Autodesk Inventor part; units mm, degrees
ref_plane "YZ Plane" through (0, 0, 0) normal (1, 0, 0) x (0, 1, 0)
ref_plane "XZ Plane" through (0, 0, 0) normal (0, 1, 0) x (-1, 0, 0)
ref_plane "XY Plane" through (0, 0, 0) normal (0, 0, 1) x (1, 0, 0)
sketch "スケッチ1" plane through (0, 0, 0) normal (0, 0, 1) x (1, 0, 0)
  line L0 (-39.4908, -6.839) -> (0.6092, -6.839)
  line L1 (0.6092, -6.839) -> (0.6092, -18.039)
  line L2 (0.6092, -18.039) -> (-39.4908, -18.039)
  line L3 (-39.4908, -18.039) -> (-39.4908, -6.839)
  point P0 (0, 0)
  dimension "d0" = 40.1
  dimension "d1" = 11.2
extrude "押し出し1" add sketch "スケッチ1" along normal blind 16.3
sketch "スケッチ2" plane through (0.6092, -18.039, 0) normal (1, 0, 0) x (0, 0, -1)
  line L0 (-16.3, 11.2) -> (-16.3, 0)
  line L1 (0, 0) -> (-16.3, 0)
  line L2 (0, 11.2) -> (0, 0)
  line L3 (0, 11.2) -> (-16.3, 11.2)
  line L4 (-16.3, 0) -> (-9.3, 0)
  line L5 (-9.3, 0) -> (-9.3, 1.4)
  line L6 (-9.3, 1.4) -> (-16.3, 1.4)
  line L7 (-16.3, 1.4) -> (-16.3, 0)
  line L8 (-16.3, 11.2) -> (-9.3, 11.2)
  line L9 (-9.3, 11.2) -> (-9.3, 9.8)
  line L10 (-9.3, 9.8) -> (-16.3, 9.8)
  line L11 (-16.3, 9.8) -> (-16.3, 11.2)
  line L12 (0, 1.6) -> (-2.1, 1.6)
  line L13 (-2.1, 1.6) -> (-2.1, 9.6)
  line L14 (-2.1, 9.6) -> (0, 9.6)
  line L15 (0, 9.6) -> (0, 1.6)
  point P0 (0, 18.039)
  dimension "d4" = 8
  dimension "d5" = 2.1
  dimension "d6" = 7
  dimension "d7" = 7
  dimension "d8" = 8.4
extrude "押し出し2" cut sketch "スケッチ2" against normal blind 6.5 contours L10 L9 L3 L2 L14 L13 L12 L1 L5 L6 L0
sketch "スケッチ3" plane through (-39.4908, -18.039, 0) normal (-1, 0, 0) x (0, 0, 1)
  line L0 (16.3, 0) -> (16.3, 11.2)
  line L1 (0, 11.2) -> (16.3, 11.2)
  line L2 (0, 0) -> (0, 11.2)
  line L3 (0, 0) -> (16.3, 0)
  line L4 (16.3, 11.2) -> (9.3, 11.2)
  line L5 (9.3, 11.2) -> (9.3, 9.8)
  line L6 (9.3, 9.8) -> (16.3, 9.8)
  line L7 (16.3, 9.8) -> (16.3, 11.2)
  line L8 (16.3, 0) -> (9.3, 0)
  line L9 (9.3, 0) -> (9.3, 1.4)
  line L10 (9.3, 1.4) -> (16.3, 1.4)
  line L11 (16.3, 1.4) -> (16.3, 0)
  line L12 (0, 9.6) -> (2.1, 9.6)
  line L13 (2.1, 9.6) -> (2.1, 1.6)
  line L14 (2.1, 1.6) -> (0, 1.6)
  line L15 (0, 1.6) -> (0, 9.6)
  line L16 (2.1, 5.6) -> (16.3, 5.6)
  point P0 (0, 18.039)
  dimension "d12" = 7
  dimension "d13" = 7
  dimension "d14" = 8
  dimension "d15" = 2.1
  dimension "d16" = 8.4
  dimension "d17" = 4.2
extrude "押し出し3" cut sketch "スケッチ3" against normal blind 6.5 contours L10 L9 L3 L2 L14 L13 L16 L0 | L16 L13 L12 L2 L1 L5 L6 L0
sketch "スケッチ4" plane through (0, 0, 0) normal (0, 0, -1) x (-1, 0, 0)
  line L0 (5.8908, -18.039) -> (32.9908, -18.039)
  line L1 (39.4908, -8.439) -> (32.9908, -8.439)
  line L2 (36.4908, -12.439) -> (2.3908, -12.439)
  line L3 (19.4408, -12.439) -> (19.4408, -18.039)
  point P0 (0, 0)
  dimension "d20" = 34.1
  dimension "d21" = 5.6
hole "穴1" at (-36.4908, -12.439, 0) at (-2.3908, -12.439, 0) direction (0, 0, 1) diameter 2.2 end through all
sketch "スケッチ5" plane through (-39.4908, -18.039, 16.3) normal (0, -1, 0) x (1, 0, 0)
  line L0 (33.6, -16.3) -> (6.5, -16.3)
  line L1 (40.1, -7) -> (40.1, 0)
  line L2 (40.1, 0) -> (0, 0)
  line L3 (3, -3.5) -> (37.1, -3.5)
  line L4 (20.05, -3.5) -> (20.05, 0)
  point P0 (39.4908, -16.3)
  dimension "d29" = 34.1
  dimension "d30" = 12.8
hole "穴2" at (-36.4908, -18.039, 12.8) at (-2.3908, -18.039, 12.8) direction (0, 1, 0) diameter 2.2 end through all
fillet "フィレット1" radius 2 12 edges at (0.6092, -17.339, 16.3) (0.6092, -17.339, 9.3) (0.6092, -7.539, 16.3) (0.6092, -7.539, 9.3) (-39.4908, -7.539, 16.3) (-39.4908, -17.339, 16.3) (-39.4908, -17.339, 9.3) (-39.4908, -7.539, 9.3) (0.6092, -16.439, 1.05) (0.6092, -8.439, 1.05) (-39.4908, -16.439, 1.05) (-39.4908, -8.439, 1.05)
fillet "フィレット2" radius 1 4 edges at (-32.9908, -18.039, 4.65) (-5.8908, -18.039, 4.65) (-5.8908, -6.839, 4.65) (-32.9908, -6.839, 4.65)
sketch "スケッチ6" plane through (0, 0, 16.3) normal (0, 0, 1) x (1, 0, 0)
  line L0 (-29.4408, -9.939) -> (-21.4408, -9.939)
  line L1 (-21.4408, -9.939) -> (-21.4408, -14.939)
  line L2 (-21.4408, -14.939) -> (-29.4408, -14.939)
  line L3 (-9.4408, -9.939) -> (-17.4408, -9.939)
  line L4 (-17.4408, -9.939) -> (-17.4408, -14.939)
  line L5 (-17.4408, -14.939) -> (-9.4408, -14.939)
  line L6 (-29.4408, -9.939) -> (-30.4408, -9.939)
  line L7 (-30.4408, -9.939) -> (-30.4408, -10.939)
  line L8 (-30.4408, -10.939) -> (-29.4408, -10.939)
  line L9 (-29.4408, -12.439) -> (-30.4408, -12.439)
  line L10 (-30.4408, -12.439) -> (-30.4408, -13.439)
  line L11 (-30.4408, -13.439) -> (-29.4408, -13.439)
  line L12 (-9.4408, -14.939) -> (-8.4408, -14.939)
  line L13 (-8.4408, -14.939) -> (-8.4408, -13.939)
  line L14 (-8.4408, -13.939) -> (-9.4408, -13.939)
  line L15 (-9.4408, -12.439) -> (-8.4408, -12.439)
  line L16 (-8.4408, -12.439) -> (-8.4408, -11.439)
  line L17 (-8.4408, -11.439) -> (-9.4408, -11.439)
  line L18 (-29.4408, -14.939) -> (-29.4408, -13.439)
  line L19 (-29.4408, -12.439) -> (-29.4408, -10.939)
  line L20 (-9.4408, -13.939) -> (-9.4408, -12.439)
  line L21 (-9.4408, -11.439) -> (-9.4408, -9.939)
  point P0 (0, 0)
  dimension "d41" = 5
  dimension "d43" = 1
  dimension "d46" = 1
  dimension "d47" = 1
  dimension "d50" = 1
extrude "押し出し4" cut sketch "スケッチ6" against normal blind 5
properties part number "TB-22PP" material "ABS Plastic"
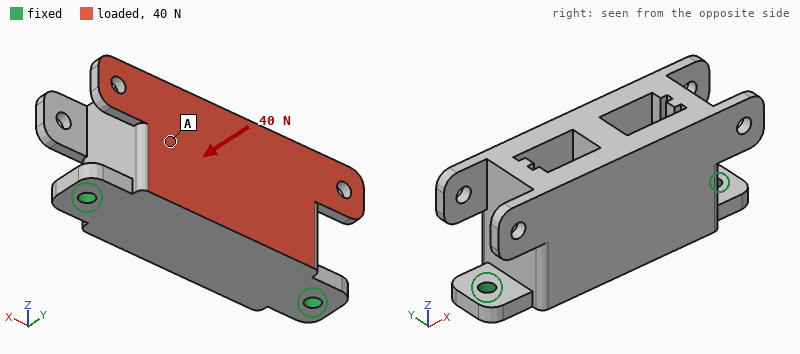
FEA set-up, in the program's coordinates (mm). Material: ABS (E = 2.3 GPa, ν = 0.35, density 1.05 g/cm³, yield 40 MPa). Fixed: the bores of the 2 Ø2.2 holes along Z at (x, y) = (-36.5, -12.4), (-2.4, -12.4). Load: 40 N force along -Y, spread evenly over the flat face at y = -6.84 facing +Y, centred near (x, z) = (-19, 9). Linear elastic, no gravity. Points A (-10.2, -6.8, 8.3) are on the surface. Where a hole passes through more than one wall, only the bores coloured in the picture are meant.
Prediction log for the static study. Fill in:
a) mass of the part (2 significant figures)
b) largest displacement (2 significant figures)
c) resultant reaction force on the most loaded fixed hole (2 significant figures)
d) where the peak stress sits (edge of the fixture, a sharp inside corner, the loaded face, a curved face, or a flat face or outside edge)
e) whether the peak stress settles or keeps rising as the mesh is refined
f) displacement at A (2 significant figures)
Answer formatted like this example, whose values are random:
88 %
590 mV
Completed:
5.2 g
0.44 mm
20 N
edge of the fixture
keeps rising
0.24 mm
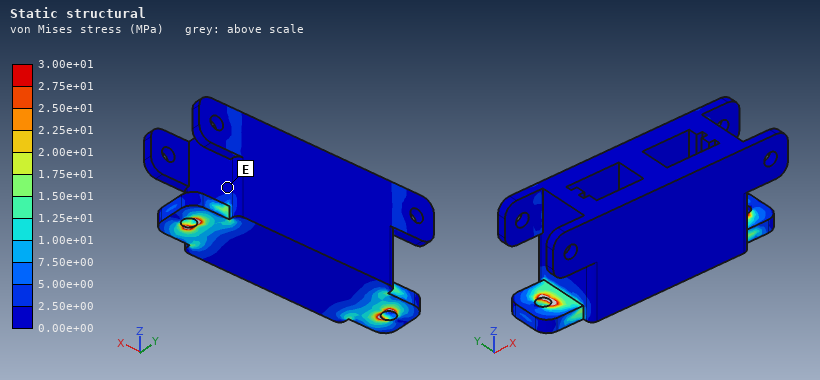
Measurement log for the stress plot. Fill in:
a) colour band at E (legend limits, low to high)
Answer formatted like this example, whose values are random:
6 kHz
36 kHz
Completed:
0.00e+00 to 2.50e+00 MPa
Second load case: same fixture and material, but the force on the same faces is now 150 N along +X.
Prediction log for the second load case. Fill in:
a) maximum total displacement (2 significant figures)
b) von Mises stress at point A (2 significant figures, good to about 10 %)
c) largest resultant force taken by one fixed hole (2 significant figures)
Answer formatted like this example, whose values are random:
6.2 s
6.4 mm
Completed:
0.11 mm
1.9 MPa
89 N
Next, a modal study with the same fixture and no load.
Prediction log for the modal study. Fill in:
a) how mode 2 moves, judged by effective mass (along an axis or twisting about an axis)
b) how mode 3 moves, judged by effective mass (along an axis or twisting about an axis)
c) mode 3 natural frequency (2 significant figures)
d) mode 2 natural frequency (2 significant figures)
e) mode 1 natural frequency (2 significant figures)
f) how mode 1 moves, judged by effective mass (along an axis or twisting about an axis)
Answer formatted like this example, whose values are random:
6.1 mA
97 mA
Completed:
along Z
along X
4200 Hz
3400 Hz
890 Hz
along Y
